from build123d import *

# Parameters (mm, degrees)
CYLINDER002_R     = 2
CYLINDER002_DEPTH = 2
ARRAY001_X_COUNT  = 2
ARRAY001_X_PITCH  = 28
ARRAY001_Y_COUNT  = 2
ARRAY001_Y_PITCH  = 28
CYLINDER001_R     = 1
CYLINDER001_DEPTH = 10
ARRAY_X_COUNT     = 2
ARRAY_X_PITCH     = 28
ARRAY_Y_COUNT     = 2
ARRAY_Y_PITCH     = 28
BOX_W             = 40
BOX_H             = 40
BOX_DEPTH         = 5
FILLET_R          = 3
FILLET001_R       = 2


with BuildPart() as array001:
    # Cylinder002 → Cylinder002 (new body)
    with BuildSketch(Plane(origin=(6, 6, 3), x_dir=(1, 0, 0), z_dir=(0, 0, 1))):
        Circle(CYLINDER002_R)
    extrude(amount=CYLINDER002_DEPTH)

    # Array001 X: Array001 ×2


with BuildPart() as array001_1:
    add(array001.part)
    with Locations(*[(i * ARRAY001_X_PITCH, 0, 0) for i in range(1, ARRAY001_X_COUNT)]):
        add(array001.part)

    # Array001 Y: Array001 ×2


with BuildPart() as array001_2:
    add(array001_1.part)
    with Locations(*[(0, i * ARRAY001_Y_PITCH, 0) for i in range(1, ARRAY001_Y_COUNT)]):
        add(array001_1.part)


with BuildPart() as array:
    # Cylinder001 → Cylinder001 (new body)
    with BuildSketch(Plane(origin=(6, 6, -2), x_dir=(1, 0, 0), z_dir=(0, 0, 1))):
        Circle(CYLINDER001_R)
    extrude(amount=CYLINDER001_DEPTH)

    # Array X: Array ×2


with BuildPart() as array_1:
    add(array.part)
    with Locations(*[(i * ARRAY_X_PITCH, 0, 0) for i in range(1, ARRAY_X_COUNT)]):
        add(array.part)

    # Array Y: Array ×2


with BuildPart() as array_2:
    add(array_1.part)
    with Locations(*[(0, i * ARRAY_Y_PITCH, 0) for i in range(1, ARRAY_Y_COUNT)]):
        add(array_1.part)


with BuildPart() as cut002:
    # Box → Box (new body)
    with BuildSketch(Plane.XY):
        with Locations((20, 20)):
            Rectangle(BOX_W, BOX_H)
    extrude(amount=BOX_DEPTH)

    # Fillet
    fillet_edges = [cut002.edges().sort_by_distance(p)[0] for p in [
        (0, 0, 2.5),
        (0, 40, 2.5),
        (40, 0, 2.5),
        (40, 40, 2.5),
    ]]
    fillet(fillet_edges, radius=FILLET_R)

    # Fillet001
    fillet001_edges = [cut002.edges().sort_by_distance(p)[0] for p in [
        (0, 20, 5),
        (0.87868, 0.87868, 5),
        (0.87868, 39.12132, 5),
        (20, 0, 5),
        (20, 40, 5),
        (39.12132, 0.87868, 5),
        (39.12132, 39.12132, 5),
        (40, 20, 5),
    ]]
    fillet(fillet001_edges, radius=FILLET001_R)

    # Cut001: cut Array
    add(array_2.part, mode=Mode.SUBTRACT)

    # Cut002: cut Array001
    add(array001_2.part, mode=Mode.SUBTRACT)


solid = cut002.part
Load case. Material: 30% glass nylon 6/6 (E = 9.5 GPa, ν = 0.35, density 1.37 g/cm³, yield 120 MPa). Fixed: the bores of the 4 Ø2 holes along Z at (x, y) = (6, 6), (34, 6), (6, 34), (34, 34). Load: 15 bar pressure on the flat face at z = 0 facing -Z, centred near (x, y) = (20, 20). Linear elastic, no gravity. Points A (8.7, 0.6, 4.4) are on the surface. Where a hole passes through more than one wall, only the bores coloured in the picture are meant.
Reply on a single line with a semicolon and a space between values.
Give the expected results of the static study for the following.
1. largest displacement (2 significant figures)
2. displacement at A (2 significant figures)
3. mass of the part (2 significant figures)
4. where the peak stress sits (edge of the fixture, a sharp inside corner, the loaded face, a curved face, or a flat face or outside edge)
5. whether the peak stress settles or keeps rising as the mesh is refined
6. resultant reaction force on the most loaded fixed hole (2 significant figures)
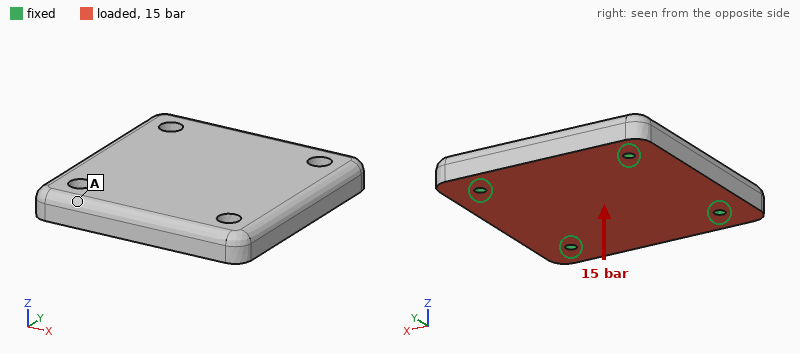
0.11 mm; 0.017 mm; 11 g; edge of the fixture; keeps rising; 630 N
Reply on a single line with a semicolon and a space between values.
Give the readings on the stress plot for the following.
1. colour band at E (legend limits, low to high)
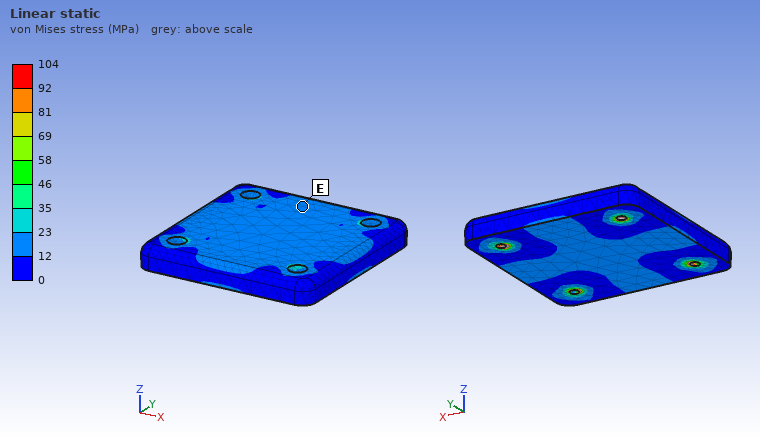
12 to 23 MPa
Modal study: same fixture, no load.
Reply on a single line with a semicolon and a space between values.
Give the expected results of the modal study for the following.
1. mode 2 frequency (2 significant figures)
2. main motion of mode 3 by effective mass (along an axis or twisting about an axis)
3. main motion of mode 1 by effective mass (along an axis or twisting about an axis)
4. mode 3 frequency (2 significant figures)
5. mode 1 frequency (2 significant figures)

11 kHz; twisting about Y; along Z; 12 kHz; 8300 Hz
